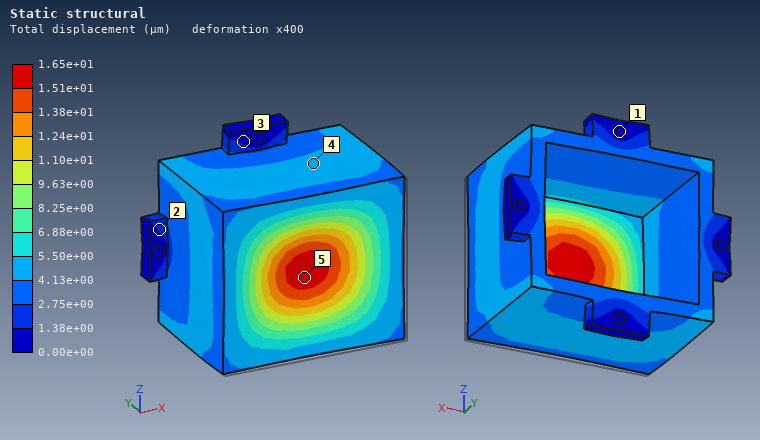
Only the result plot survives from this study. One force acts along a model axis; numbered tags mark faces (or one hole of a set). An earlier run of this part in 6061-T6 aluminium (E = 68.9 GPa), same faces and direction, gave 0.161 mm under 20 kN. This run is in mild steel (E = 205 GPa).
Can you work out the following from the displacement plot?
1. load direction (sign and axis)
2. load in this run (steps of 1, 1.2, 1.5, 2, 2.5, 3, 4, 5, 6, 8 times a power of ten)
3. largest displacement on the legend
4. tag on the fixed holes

+Y
6 kN
1.65e+01 µm
1
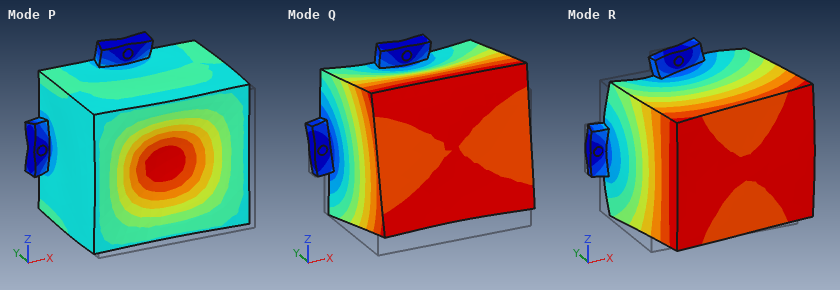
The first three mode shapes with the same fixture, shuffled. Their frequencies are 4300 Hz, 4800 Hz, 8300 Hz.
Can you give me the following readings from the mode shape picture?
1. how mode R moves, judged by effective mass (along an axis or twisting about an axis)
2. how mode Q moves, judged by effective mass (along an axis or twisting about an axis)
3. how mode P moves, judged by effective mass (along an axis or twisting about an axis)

along X
along Z
along Y
